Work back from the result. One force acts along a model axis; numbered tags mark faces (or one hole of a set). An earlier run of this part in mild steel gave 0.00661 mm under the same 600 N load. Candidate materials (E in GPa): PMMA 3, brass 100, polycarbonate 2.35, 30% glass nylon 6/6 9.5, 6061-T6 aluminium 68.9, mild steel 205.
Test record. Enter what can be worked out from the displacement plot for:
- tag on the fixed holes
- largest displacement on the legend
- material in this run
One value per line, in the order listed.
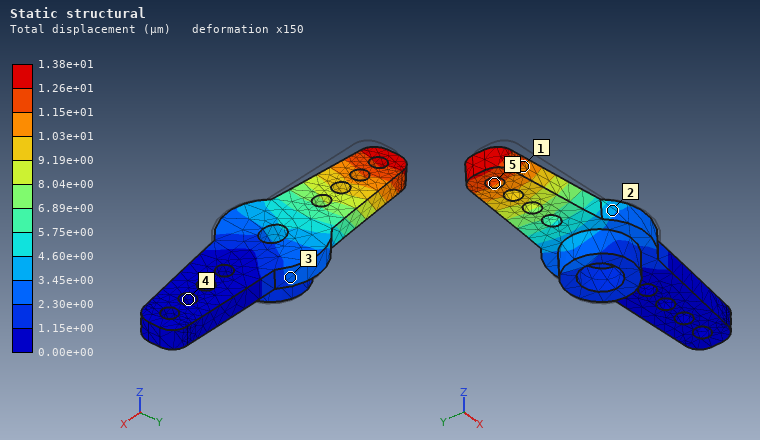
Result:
4
1.38e+01 µm
brass
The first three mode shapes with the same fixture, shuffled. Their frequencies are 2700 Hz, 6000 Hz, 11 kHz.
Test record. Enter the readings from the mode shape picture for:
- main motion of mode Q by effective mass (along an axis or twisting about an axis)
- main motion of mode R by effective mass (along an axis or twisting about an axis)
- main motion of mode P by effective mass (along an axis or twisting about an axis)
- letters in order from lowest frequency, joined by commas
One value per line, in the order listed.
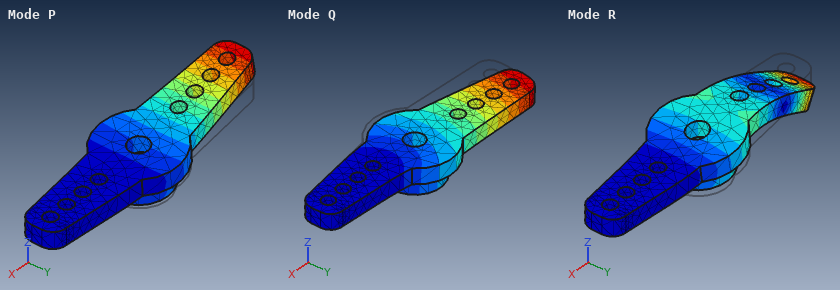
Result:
along Y
along Z
along Z
P, Q, R
